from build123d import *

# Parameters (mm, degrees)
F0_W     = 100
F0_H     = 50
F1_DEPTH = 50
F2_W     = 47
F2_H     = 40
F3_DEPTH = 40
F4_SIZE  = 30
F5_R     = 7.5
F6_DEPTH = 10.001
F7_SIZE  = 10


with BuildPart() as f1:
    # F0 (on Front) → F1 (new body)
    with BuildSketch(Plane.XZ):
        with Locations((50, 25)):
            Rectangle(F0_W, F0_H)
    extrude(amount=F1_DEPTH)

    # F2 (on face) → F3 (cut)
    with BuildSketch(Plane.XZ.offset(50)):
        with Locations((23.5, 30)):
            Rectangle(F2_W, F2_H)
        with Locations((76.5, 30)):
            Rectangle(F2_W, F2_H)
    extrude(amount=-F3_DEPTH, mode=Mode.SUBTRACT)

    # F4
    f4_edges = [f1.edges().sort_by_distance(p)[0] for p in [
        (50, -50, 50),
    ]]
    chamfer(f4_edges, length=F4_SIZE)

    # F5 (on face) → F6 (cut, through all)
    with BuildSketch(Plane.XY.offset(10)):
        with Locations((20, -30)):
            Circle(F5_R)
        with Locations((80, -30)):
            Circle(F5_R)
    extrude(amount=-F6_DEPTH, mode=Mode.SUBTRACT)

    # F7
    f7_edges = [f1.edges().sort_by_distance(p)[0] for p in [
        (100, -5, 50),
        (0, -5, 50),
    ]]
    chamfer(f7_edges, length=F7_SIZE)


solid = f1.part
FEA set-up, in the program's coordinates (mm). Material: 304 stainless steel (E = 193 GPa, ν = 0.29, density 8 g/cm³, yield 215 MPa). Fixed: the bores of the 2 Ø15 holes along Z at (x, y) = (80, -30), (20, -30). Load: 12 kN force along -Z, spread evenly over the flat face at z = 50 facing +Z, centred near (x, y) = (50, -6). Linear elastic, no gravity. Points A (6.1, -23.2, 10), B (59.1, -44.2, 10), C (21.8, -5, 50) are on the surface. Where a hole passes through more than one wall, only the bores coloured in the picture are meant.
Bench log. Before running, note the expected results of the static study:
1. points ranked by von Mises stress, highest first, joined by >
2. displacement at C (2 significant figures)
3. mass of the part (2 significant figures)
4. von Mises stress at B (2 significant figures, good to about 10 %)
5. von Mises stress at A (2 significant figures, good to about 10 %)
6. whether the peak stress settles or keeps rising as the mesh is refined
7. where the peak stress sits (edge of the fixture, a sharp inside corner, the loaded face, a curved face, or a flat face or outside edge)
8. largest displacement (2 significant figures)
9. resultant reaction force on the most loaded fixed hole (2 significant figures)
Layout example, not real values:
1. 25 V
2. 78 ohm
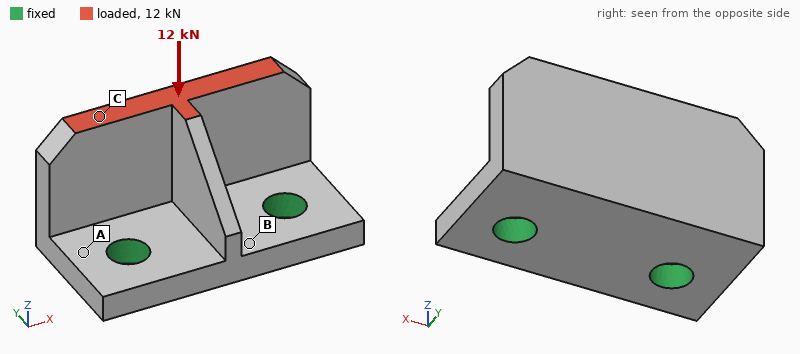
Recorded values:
1. A > B > C
2. 58 µm
3. 740 g
4. 33 MPa
5. 60 MPa
6. keeps rising
7. edge of the fixture
8. 63 µm
9. 6.0 kN
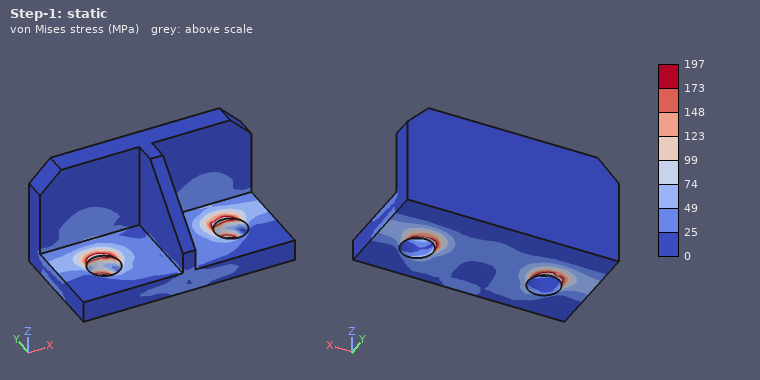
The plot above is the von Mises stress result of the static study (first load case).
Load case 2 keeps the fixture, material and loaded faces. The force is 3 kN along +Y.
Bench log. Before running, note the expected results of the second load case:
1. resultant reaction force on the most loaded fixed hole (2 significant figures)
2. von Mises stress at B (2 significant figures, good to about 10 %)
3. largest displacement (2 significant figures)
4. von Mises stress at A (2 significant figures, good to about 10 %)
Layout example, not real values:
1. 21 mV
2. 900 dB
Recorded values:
1. 1.5 kN
2. 32 MPa
3. 56 µm
4. 30 MPa
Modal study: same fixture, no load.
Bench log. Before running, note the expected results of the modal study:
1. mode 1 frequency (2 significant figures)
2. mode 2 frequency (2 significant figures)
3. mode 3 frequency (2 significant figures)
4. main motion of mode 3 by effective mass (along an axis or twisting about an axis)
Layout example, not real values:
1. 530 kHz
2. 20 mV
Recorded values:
1. 3100 Hz
2. 4200 Hz
3. 6500 Hz
4. along X
